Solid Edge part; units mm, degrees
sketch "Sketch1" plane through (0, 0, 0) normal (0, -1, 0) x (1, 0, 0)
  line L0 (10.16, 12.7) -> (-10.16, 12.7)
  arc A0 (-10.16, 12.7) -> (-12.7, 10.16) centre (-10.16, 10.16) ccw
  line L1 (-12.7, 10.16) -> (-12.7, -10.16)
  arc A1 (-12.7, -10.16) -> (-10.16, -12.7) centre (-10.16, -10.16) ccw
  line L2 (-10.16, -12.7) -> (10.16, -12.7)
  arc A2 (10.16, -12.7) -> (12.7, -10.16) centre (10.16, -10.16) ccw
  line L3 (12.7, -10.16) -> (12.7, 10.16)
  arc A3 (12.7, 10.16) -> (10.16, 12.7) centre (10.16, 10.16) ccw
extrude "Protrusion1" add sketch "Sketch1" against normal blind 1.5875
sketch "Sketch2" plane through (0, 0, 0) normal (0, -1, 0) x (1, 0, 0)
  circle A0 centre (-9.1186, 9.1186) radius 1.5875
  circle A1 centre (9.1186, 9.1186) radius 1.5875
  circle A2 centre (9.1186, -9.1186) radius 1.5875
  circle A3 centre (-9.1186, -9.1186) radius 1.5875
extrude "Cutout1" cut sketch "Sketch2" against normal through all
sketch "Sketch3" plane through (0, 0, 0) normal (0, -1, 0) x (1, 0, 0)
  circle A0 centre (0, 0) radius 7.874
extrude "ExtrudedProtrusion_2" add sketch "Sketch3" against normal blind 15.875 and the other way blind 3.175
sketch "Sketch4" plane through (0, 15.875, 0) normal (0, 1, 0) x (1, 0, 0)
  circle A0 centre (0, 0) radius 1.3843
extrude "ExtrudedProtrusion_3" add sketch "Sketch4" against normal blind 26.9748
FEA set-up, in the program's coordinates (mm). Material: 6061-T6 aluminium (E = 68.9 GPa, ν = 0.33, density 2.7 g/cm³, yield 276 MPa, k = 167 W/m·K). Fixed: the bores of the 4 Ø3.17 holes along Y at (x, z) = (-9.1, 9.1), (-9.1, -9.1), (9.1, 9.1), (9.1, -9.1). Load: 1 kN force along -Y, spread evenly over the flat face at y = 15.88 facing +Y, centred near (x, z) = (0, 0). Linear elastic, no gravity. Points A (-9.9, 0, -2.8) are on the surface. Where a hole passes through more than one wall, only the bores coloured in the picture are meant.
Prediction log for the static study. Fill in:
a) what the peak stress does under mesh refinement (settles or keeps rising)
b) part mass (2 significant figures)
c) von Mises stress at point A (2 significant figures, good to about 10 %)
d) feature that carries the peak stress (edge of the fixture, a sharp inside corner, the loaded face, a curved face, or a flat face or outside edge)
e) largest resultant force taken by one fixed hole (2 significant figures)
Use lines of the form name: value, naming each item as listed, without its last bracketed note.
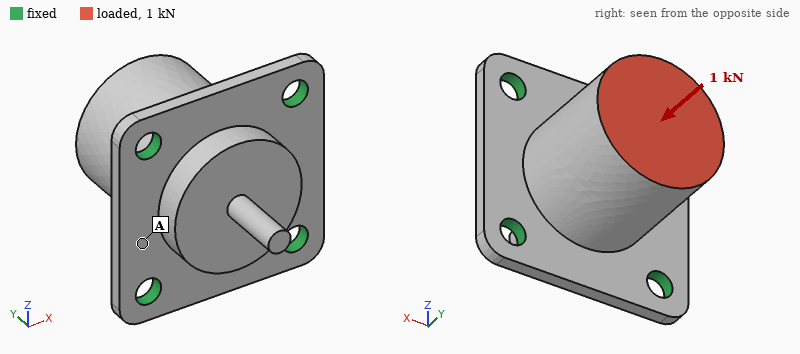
what the peak stress does under mesh refinement: keeps rising
part mass: 12 g
von Mises stress at point A: 28 MPa
feature that carries the peak stress: edge of the fixture
largest resultant force taken by one fixed hole: 250 N
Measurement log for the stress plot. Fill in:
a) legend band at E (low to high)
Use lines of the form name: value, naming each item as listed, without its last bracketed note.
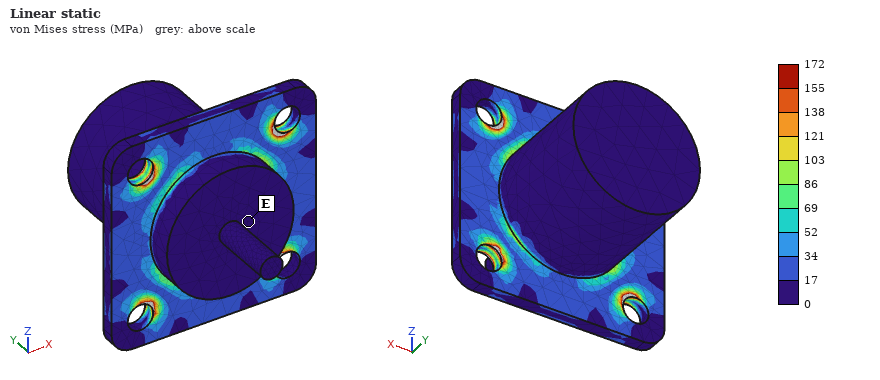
legend band at E: 0 to 17 MPa
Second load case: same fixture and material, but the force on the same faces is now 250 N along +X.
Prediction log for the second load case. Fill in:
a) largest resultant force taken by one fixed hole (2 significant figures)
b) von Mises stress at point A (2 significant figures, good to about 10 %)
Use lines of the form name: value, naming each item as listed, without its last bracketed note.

largest resultant force taken by one fixed hole: 140 N
von Mises stress at point A: 20 MPa
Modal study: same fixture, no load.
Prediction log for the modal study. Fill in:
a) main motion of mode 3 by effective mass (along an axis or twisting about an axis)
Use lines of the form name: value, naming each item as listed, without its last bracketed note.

main motion of mode 3 by effective mass: along Y
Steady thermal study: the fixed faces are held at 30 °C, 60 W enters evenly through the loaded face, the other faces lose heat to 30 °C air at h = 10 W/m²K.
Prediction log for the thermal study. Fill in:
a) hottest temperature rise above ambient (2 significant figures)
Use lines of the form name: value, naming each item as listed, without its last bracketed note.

hottest temperature rise above ambient: 57 K
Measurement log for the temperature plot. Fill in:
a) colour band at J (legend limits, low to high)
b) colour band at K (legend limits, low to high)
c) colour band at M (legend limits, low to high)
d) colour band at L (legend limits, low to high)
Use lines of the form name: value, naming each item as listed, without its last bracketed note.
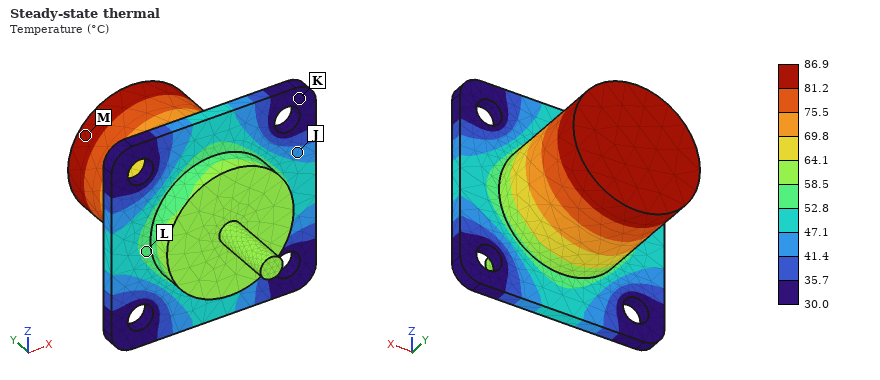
colour band at J: 41.4 to 47.1 °C
colour band at K: 30.0 to 35.7 °C
colour band at M: 81.2 to 86.9 °C
colour band at L: 52.8 to 58.5 °C
